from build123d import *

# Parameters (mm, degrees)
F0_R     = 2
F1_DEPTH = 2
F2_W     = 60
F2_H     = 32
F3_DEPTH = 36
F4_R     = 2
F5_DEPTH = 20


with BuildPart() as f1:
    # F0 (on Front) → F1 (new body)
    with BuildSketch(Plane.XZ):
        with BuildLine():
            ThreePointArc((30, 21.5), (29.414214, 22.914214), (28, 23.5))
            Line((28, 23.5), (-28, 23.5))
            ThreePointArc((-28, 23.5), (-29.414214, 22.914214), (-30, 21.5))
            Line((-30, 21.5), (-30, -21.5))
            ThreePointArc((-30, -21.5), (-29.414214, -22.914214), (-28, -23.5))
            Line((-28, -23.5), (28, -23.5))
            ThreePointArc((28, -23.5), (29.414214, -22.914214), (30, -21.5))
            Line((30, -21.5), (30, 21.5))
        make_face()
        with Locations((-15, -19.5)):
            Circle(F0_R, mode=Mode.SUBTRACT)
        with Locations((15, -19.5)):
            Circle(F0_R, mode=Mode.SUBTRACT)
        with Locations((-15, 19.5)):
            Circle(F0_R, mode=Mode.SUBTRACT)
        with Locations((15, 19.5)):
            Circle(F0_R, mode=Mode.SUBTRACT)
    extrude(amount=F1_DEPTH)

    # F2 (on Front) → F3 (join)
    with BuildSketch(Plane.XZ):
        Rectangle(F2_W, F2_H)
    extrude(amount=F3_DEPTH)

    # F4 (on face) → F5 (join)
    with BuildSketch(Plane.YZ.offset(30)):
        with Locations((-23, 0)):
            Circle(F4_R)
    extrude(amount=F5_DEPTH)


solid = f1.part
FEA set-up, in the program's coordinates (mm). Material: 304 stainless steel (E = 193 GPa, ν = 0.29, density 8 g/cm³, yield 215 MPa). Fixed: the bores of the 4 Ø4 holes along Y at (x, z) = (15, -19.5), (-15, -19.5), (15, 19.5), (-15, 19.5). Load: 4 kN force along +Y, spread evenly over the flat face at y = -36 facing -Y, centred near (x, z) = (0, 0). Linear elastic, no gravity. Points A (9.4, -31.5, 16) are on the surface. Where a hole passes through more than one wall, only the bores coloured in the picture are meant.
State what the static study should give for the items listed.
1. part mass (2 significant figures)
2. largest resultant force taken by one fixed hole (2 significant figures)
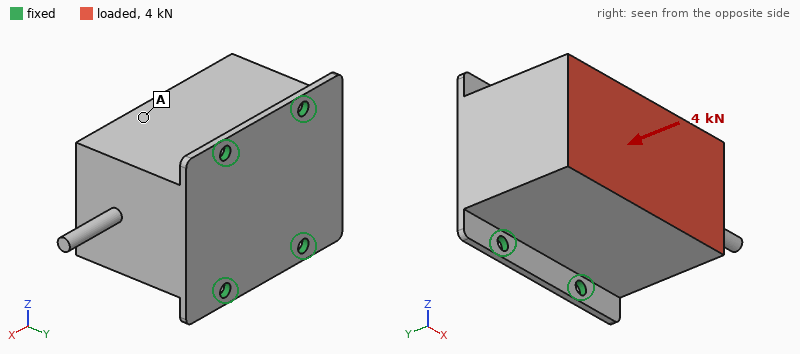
570 g
1.1 kN
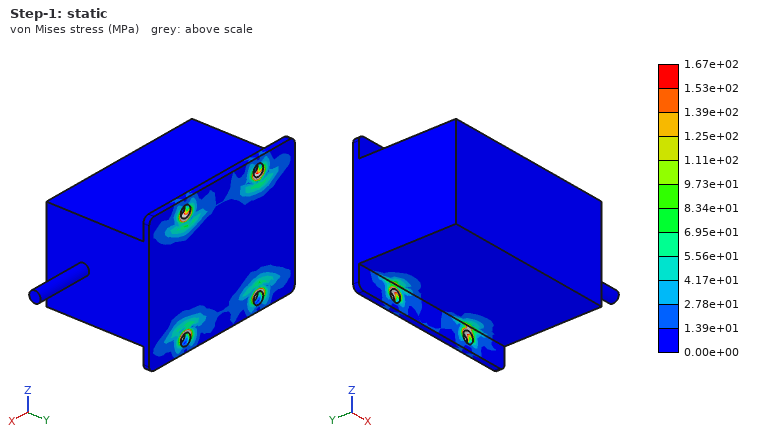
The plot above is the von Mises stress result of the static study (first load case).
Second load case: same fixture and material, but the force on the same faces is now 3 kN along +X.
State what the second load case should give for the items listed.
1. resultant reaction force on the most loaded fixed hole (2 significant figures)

2.0 kN
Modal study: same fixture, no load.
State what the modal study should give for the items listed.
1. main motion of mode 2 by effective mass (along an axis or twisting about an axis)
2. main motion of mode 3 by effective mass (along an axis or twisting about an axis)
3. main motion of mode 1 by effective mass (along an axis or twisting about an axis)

along Z
along Y
along X
